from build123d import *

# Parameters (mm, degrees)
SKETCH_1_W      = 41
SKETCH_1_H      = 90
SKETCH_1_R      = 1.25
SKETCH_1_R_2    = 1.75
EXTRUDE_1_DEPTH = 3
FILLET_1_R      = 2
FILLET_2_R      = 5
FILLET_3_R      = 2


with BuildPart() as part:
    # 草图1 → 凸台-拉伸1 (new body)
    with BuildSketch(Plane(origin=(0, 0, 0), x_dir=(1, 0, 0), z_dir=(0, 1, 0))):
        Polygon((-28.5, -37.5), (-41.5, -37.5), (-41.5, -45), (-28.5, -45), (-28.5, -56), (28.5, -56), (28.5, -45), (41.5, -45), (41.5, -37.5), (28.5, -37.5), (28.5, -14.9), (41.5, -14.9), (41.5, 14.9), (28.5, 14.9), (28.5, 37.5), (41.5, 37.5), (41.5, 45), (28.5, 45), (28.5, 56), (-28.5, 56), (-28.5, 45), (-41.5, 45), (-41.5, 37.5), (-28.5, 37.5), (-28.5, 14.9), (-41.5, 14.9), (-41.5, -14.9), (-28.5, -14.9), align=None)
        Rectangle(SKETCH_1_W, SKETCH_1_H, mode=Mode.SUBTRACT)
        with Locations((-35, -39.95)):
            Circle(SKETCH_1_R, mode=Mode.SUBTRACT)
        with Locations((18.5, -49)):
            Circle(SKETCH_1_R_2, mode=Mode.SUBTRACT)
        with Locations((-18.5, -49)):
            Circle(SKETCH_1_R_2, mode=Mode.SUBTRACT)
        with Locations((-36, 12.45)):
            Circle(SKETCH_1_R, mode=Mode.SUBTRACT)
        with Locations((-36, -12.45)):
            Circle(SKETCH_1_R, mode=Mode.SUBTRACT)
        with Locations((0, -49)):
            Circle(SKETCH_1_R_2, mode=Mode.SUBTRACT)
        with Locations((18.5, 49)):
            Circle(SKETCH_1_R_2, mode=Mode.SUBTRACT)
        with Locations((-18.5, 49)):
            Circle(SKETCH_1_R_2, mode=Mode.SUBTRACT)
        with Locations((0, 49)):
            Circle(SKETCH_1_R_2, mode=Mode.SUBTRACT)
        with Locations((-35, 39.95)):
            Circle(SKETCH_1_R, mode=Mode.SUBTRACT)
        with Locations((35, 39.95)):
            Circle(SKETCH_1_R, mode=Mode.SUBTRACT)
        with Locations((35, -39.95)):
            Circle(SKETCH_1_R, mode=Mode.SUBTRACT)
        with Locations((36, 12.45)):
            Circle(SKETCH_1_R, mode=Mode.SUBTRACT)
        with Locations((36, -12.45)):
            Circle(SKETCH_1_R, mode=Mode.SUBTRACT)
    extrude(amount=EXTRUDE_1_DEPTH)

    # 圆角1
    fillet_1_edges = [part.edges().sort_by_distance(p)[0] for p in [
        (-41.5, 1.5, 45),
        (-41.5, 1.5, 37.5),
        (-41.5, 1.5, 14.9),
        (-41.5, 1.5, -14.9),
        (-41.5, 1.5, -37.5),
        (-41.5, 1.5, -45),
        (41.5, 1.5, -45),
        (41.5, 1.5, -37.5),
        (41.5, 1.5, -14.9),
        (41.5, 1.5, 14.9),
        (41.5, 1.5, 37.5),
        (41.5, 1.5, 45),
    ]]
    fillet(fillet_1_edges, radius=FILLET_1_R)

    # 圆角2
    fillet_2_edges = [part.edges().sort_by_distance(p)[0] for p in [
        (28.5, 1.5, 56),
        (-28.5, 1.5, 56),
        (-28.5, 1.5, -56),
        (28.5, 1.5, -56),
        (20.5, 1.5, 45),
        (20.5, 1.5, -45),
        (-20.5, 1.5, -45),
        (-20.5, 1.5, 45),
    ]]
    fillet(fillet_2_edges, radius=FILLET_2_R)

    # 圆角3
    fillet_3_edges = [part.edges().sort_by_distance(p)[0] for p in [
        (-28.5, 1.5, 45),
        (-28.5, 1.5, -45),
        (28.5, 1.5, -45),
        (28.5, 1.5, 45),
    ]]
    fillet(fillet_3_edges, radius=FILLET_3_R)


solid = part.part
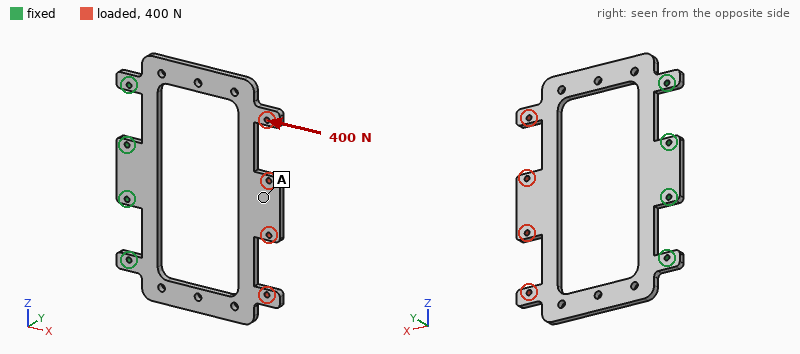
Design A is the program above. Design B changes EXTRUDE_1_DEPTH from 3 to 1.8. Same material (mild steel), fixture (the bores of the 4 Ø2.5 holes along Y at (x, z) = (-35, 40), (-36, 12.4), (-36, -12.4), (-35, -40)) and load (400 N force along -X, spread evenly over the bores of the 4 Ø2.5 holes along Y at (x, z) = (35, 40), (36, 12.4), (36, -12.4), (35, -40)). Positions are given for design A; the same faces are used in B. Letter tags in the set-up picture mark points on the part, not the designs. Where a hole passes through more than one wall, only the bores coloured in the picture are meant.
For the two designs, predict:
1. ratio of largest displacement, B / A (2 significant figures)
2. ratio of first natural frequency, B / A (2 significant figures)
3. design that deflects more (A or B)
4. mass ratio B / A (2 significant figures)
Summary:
1.7
0.61
B
0.60
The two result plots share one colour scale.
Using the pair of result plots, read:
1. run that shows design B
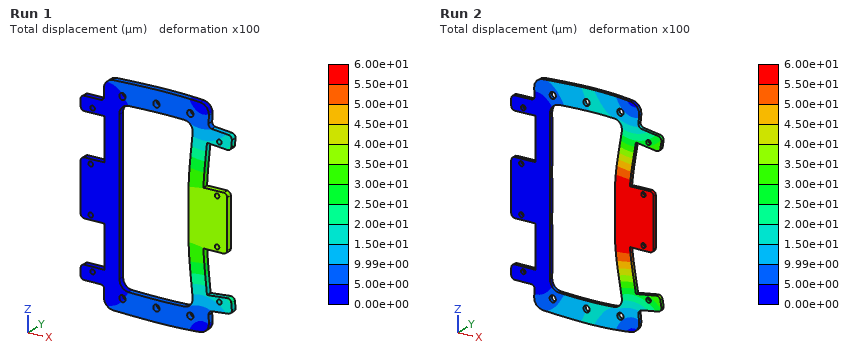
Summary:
Run 2
